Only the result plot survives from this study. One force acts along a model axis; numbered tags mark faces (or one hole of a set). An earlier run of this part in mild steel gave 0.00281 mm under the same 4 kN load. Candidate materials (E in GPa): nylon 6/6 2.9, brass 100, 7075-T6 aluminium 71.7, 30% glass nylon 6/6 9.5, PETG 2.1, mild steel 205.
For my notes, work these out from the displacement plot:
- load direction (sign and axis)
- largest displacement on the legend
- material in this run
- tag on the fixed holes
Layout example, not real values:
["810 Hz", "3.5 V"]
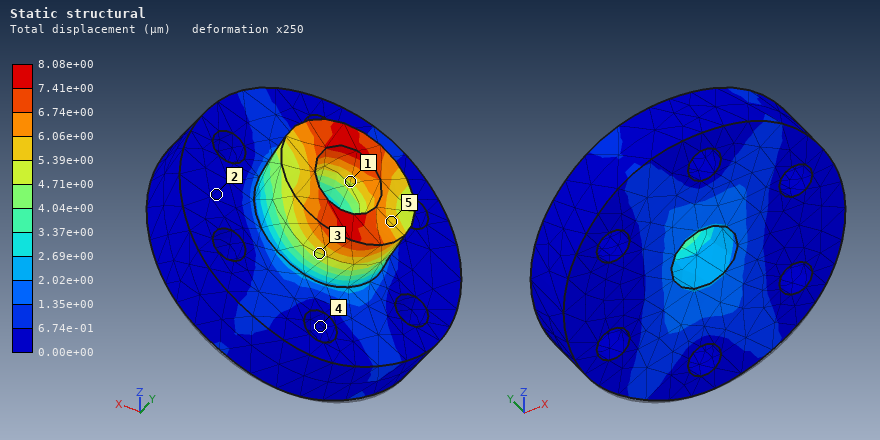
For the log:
["+Z", "8.08e+00 µm", "7075-T6 aluminium", "4"]
